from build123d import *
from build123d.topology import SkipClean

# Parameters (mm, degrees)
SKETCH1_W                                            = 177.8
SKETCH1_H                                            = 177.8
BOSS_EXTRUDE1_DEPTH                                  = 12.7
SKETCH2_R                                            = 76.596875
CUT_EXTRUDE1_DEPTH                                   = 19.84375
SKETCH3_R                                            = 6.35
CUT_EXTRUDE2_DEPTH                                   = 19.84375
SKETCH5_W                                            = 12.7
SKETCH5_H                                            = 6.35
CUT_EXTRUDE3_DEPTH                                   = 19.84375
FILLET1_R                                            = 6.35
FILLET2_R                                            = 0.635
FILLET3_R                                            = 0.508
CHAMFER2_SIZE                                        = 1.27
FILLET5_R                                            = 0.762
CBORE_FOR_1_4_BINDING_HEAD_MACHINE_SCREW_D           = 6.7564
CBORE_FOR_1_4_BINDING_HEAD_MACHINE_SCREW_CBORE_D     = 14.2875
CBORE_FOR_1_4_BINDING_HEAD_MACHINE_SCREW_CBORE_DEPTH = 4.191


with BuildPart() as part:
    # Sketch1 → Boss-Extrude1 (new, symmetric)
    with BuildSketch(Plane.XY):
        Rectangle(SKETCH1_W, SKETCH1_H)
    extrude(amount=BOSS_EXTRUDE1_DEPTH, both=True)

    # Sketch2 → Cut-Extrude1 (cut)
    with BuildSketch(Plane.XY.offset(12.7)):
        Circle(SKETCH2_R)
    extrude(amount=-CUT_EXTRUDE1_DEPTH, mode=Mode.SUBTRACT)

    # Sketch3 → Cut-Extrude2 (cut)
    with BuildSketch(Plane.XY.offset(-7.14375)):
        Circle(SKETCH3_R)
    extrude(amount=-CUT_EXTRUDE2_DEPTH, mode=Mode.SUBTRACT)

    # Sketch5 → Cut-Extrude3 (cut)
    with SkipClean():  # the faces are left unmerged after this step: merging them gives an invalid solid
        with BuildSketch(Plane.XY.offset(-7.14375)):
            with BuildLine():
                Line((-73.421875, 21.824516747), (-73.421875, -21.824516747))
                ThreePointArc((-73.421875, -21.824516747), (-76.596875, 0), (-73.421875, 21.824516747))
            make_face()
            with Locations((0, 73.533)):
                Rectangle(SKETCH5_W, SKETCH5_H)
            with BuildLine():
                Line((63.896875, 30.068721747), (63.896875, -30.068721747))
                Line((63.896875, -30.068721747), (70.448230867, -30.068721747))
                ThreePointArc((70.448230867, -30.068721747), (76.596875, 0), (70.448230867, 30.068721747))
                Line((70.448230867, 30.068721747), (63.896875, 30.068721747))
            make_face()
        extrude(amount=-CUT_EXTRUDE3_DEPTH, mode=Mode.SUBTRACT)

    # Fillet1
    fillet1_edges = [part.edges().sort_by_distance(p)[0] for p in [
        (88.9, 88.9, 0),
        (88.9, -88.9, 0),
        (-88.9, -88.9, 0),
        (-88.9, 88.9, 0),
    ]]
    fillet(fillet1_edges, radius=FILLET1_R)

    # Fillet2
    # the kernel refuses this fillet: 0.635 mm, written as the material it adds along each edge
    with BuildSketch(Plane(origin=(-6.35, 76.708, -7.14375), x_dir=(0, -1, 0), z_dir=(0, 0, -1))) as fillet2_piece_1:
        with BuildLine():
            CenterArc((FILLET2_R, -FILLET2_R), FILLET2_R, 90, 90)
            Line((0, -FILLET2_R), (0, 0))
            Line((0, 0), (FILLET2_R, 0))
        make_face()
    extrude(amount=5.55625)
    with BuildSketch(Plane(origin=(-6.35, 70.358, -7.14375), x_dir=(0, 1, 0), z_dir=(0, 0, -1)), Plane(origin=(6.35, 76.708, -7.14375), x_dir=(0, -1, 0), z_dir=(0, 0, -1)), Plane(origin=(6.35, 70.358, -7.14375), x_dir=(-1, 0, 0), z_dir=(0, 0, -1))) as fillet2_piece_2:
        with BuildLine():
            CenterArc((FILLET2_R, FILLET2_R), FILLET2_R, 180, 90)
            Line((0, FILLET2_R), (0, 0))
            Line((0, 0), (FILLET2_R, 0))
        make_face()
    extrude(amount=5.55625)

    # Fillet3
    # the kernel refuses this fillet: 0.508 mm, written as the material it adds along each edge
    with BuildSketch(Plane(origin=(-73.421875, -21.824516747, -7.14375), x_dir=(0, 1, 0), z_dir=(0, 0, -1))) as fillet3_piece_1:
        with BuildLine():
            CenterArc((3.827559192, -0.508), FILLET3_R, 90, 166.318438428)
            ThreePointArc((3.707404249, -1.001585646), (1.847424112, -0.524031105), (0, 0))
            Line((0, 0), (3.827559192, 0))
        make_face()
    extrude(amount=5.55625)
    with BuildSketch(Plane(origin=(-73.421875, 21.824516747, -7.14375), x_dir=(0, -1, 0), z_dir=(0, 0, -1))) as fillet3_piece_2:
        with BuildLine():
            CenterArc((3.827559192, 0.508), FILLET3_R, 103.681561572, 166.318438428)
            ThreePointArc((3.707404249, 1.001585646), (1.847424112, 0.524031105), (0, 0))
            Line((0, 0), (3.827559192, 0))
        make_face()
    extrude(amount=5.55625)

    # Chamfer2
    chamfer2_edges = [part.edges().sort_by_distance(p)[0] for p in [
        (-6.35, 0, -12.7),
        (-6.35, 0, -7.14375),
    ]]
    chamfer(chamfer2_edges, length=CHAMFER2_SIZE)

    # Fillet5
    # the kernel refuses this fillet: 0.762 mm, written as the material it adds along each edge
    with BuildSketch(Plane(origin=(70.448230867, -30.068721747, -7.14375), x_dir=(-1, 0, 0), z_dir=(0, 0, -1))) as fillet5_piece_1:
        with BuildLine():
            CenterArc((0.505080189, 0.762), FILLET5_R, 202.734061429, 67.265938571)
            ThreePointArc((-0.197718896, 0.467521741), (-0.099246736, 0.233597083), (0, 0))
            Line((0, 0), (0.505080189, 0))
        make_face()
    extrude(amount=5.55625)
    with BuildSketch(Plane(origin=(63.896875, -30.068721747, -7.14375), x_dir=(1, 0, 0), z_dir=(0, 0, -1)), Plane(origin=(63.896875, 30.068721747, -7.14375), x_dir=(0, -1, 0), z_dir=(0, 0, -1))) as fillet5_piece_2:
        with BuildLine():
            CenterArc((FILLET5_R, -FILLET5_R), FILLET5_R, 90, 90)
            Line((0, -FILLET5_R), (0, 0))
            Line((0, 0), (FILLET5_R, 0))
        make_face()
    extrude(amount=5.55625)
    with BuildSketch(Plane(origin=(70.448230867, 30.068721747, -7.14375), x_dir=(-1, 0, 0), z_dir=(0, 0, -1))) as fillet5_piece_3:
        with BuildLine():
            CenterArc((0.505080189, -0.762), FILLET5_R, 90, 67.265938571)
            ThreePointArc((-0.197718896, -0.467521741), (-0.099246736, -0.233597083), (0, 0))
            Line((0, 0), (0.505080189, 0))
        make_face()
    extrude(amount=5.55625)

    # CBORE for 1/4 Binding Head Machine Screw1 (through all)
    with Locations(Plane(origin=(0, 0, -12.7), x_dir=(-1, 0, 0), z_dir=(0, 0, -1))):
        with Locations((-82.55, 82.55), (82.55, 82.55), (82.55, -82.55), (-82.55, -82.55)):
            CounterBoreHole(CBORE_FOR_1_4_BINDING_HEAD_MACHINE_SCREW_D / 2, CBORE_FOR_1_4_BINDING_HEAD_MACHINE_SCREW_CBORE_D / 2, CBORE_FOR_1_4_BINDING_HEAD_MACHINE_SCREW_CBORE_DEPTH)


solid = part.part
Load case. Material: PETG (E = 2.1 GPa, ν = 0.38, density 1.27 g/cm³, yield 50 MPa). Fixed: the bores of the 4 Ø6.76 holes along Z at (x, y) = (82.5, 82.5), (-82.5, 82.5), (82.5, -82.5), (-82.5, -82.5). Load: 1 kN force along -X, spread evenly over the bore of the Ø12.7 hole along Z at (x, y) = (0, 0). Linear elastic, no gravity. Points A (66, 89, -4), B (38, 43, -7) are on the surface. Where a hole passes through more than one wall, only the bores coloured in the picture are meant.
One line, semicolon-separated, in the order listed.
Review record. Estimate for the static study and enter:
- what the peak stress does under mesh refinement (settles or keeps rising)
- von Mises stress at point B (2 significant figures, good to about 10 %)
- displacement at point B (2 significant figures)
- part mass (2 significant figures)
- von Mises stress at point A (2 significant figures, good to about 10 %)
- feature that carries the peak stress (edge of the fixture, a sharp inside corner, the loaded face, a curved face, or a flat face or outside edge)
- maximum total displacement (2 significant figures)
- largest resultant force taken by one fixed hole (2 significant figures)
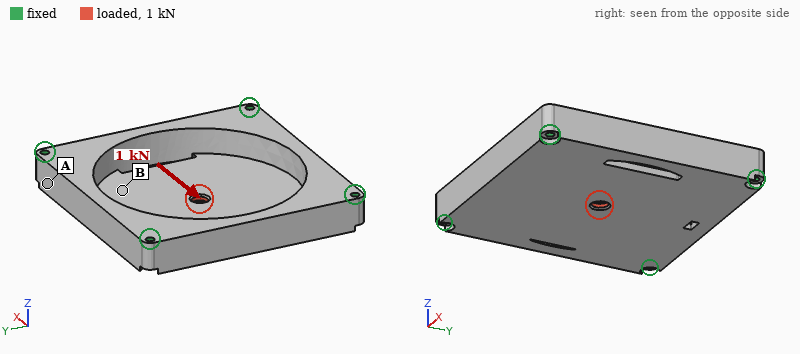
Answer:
keeps rising; 1.2 MPa; 40 µm; 540 g; 0.54 MPa; a sharp inside corner; 95 µm; 290 N
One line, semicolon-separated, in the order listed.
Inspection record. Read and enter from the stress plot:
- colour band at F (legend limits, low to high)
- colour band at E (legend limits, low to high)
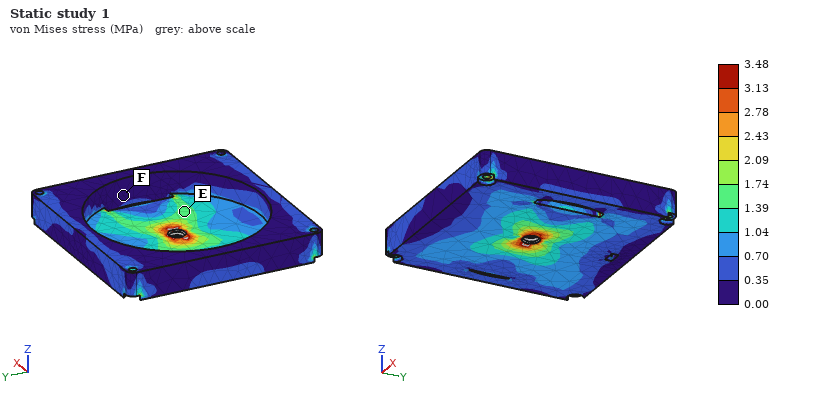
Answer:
0.00 to 0.35 MPa; 1.39 to 1.74 MPa
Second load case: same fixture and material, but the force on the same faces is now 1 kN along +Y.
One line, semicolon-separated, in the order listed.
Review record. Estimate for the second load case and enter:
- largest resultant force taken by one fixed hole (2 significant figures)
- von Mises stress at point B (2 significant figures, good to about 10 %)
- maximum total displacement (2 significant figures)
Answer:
300 N; 1.2 MPa; 97 µm
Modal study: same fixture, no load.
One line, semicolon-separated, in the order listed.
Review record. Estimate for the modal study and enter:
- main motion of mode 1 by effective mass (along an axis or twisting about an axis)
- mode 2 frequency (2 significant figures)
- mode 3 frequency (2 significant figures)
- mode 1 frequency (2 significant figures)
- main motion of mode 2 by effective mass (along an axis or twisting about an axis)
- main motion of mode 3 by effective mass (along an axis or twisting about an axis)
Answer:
along Z; 810 Hz; 850 Hz; 480 Hz; twisting about Y; twisting about X
